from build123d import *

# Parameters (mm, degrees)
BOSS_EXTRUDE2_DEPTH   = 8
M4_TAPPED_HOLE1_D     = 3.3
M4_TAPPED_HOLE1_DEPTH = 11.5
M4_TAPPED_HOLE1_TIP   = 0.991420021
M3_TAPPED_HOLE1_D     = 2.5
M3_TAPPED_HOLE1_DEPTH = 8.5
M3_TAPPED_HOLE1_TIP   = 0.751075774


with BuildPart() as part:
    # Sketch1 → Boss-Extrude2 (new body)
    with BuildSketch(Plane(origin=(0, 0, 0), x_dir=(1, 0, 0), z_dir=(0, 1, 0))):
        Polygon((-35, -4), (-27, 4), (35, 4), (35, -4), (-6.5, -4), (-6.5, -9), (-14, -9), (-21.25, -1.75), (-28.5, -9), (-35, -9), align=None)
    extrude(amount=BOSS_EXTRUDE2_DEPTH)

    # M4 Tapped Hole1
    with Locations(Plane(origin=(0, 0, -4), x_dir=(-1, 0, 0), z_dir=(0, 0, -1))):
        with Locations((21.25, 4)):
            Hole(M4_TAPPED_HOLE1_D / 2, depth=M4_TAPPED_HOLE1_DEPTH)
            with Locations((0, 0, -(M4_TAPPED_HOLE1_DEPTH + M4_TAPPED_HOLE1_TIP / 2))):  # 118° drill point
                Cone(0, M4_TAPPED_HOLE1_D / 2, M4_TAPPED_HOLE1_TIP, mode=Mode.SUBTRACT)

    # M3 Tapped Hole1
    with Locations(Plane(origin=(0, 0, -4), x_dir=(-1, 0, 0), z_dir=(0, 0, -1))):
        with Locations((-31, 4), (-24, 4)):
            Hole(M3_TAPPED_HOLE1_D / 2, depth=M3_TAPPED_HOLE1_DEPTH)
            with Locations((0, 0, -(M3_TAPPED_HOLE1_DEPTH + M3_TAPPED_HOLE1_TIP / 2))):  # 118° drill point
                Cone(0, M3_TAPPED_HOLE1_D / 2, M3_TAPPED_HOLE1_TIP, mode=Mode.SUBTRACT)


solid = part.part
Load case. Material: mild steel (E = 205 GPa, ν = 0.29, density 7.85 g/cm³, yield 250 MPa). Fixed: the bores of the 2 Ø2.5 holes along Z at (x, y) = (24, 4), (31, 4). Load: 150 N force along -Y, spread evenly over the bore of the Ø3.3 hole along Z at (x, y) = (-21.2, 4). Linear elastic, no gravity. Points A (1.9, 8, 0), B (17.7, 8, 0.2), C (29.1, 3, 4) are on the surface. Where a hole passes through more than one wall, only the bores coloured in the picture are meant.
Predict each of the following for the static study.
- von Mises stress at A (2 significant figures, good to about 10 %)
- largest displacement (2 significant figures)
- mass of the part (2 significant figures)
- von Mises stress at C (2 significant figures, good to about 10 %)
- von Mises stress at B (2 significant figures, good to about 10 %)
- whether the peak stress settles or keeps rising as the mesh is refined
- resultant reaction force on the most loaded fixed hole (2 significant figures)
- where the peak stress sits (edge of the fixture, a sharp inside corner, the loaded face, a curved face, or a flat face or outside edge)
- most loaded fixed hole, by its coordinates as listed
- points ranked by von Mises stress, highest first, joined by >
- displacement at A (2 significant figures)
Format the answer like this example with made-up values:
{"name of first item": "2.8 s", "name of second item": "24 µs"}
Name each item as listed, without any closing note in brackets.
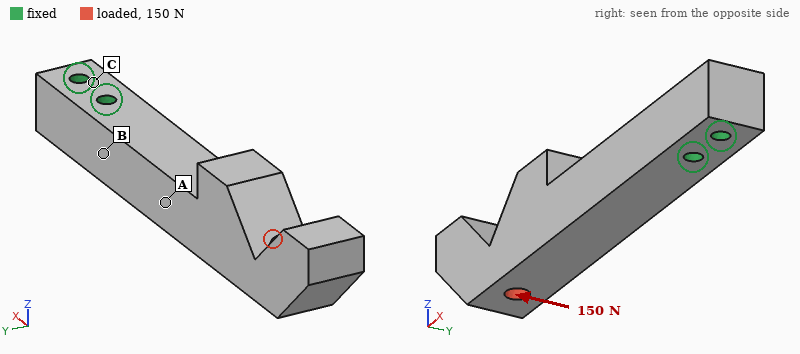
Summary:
{"von Mises stress at A": "41 MPa", "largest displacement": "0.11 mm", "mass of the part": "38 g", "von Mises stress at C": "21 MPa", "von Mises stress at B": "69 MPa", "whether the peak stress settles or keeps rising as the mesh is refined": "keeps rising", "resultant reaction force on the most loaded fixed hole": "610 N", "where the peak stress sits": "edge of the fixture", "most loaded fixed hole, by its coordinates as listed": "(24, 4)", "points ranked by von Mises stress, highest first, joined by >": "B > A > C", "displacement at A": "0.026 mm"}
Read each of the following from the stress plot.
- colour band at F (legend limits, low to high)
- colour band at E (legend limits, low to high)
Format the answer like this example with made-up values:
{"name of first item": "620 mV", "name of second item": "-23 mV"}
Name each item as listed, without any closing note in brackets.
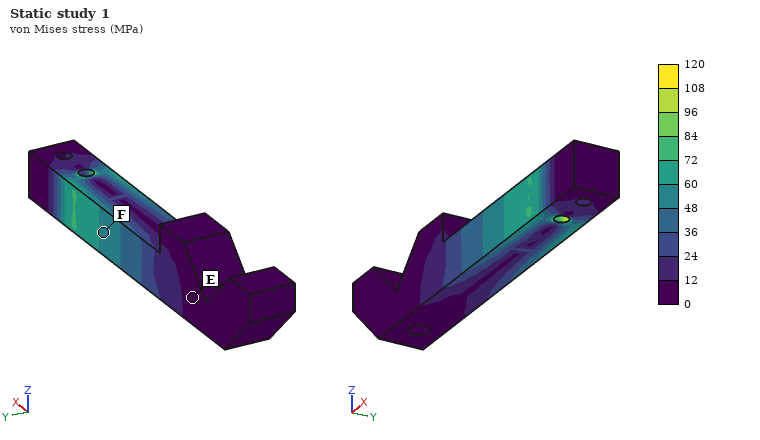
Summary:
{"colour band at F": "48 to 60 MPa", "colour band at E": "0 to 12 MPa"}
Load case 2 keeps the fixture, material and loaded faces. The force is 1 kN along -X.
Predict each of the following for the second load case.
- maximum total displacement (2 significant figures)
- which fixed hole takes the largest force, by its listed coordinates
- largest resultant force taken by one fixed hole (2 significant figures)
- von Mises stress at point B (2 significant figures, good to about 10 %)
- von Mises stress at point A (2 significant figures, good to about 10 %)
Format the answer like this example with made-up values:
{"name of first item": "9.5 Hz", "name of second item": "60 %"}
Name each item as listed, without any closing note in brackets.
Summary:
{"maximum total displacement": "14 µm", "which fixed hole takes the largest force, by its listed coordinates": "(24, 4)", "largest resultant force taken by one fixed hole": "880 N", "von Mises stress at point B": "15 MPa", "von Mises stress at point A": "16 MPa"}
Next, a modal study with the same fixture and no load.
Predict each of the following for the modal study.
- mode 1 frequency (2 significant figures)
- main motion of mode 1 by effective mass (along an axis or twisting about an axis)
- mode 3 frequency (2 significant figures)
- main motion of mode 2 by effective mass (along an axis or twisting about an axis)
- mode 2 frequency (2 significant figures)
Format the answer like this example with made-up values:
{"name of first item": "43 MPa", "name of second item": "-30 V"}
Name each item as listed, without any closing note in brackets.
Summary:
{"mode 1 frequency": "1700 Hz", "main motion of mode 1 by effective mass": "along Y", "mode 3 frequency": "9100 Hz", "main motion of mode 2 by effective mass": "along Z", "mode 2 frequency": "1800 Hz"}
